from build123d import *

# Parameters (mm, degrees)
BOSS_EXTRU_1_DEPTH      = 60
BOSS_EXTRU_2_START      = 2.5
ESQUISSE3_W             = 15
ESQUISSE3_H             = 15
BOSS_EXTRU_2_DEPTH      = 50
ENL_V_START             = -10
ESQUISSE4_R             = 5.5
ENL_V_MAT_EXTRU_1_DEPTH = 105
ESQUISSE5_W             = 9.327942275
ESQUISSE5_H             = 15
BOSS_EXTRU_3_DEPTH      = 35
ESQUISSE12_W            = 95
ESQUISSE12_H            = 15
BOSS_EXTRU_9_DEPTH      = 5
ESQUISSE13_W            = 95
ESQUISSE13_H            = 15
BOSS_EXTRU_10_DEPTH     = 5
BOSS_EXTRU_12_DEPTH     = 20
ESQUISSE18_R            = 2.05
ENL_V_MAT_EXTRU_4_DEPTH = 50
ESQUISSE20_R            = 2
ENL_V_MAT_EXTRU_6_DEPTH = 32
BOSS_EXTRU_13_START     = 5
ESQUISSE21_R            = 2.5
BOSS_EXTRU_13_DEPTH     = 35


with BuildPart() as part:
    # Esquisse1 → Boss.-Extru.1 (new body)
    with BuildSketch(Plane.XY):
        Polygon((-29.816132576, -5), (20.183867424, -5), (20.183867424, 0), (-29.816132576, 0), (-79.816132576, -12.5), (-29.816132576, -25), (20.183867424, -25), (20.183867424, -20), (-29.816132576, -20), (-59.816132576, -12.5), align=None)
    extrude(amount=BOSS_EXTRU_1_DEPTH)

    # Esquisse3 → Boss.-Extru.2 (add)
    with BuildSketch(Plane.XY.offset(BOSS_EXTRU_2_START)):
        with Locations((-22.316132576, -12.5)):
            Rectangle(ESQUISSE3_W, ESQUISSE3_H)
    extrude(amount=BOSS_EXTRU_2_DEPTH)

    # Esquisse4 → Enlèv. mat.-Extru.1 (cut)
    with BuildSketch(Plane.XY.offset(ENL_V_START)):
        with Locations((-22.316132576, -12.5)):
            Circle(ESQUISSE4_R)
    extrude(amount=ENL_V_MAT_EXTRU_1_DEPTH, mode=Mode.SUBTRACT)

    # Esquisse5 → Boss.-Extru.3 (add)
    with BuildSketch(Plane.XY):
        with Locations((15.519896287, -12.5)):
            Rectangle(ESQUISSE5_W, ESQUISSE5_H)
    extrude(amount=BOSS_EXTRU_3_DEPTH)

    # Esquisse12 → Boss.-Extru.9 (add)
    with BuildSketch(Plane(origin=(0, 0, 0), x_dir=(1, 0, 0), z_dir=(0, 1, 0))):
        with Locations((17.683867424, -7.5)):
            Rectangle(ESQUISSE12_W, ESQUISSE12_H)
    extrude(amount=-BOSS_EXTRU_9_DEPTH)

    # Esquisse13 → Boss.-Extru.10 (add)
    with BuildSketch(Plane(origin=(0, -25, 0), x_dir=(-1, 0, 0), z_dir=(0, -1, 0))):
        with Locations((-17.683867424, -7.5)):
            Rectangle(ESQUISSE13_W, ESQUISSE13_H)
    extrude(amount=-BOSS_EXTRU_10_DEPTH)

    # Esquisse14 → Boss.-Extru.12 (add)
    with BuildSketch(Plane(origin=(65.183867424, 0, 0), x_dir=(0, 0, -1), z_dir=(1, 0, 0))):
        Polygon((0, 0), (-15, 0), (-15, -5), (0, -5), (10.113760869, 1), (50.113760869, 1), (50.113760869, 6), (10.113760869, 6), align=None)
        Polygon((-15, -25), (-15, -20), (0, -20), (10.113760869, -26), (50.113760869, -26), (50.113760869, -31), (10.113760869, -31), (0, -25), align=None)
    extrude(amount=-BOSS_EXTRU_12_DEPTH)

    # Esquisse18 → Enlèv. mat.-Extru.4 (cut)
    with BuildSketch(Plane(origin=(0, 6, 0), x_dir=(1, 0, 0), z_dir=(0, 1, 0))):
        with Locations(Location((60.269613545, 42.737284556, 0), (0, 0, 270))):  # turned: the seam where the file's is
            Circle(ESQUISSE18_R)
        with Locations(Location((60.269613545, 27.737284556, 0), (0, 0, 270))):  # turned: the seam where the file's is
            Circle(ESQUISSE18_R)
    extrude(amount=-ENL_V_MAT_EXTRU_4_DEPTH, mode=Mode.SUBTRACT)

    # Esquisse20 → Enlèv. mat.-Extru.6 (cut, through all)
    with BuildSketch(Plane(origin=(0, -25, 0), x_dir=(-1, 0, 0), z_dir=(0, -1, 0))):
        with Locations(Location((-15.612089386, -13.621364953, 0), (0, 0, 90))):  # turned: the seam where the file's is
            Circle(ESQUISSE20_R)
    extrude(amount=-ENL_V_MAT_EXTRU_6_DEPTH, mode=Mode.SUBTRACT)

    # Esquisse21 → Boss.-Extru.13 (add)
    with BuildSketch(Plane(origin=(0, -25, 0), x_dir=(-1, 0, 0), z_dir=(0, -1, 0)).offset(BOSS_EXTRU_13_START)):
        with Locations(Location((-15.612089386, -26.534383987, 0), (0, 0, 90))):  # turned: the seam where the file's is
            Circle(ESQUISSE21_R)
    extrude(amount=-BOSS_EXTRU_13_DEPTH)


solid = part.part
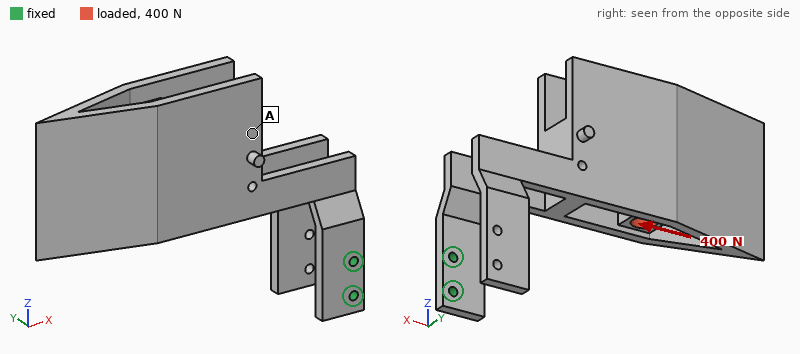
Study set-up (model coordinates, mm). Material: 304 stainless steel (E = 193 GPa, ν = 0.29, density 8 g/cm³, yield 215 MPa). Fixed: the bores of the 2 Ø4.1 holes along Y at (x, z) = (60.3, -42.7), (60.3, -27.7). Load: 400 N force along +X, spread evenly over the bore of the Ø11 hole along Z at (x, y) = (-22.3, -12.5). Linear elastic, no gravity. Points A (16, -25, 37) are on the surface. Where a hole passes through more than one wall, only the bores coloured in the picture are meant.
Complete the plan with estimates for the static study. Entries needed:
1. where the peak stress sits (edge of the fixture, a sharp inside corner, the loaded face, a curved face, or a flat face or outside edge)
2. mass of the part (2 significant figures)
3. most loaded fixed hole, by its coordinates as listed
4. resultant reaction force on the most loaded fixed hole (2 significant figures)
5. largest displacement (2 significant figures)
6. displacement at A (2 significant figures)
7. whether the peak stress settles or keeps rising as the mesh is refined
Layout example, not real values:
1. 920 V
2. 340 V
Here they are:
1. edge of the fixture
2. 650 g
3. (60.3, -27.7)
4. 1.6 kN
5. 0.91 mm
6. 0.22 mm
7. keeps rising
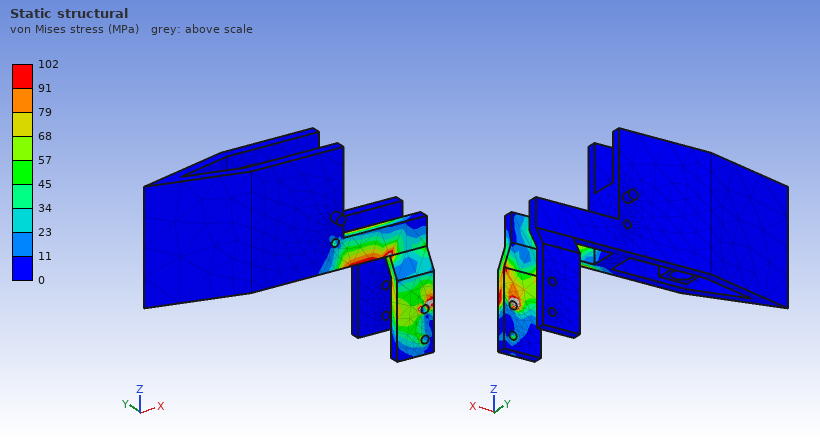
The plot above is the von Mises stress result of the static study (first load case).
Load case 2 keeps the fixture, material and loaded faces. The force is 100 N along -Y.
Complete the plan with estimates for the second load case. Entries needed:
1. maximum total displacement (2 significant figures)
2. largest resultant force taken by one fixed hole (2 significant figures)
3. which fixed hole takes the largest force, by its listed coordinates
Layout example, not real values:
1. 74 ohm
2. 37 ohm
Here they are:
1. 1.9 mm
2. 280 N
3. (60.3, -27.7)
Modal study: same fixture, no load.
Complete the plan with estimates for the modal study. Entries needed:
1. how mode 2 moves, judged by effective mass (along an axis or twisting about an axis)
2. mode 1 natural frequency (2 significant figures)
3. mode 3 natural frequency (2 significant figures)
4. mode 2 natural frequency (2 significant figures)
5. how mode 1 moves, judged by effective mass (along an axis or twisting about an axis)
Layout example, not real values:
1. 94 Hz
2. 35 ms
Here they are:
1. along Z
2. 64 Hz
3. 240 Hz
4. 170 Hz
5. along Y
